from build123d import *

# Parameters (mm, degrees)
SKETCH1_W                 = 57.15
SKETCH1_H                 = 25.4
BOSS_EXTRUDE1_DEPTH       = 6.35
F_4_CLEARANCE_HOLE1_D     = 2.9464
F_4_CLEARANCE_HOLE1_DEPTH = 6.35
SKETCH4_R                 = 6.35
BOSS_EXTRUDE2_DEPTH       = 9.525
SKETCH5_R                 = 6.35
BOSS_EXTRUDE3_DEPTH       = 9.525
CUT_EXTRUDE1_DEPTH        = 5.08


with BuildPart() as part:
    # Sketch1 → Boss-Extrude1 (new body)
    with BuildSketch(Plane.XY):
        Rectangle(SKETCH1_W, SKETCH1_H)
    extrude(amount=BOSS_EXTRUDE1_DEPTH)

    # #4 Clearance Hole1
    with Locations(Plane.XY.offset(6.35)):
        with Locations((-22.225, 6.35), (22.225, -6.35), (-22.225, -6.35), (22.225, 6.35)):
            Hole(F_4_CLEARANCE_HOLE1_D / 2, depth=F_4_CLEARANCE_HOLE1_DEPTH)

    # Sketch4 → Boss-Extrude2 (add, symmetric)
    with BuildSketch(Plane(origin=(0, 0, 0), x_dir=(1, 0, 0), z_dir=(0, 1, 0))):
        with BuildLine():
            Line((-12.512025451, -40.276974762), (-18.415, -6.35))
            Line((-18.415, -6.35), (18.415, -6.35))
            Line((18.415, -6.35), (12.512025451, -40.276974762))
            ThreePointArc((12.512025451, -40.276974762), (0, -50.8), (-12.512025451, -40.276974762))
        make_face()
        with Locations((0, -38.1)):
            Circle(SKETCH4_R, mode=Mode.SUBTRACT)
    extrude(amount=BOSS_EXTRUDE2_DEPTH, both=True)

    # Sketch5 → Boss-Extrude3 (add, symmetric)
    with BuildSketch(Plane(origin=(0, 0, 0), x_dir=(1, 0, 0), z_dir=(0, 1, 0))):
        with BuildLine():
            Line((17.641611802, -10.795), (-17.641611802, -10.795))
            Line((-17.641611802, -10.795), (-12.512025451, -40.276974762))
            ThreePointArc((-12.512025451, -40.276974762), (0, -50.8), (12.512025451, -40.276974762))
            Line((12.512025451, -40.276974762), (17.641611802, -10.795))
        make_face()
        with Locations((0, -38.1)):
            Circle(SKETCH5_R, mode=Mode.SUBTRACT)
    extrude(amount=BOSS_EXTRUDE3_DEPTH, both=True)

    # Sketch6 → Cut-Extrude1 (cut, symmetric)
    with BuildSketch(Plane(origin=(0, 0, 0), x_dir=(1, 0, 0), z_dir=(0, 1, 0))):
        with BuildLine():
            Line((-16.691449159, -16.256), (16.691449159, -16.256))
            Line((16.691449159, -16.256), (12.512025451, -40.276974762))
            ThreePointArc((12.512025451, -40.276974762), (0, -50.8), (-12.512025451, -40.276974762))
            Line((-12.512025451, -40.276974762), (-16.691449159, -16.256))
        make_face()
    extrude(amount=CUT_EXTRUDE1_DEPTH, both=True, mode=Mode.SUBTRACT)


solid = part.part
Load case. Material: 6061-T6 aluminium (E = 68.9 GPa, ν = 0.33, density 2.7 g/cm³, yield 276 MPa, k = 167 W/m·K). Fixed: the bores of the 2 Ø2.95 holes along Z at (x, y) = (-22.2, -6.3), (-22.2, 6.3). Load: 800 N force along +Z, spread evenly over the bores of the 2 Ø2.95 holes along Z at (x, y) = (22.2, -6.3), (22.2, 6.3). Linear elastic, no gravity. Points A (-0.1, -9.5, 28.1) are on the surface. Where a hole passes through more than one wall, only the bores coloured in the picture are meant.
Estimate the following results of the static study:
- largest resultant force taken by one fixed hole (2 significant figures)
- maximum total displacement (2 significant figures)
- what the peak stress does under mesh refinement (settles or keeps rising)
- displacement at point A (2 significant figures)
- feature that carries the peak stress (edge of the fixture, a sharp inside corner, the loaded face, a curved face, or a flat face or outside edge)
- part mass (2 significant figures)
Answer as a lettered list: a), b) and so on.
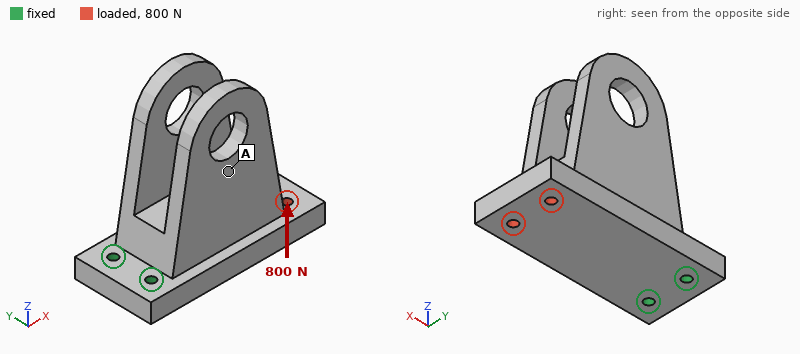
a) 410 N
b) 0.38 mm
c) keeps rising
d) 0.23 mm
e) edge of the fixture
f) 61 g
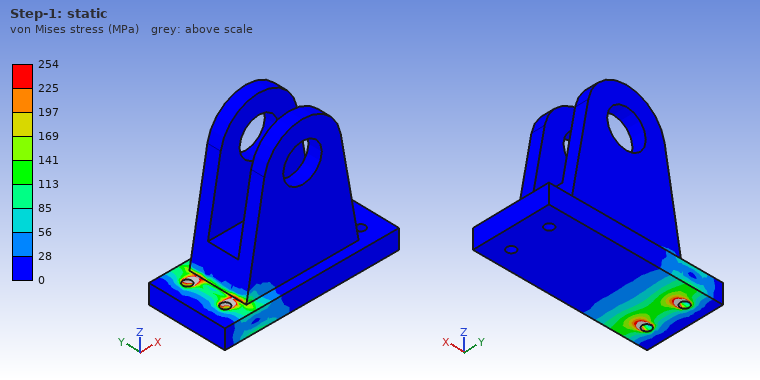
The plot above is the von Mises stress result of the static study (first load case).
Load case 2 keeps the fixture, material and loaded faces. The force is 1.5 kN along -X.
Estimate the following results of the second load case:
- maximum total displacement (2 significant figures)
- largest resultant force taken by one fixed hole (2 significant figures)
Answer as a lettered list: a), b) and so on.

a) 13 µm
b) 760 N
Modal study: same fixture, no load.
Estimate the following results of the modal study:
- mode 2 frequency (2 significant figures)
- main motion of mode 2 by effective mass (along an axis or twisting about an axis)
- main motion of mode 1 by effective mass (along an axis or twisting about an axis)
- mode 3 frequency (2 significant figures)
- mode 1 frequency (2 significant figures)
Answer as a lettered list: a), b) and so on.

a) 2800 Hz
b) along Y
c) along Z
d) 3700 Hz
e) 1500 Hz
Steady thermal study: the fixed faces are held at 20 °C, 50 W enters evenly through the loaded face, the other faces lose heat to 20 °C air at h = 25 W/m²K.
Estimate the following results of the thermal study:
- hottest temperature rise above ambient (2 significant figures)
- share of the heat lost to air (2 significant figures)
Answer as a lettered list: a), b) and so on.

a) 54 K
b) 11 %
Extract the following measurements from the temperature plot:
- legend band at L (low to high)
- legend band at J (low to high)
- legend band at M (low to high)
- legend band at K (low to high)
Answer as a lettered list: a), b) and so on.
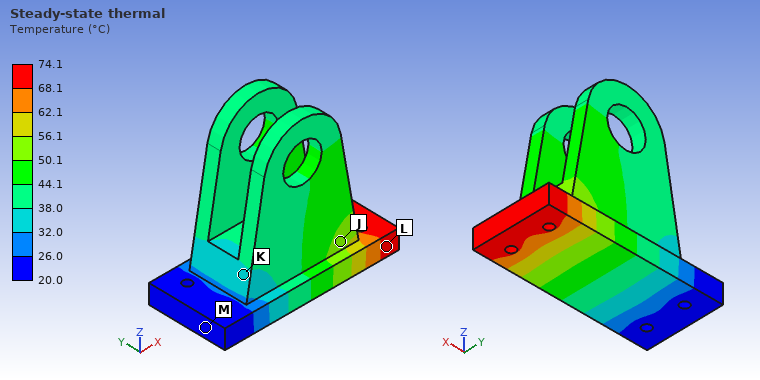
a) 68.1 to 74.1 °C
b) 50.1 to 56.1 °C
c) 20.0 to 26.0 °C
d) 32.0 to 38.0 °C
